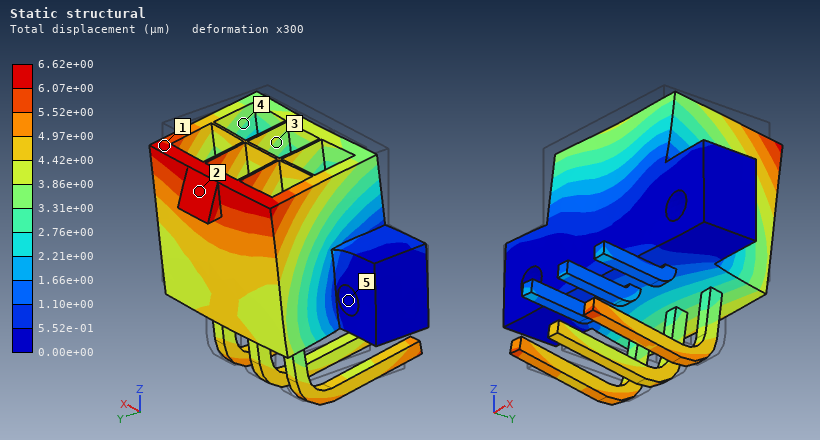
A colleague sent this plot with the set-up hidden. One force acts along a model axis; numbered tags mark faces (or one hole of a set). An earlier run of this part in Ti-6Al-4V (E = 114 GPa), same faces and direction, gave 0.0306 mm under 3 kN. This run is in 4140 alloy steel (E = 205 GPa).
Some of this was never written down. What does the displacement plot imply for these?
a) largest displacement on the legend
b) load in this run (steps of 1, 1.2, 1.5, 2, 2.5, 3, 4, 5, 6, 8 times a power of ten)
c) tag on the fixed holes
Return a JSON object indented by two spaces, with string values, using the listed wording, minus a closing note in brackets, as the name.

{
  "largest displacement on the legend": "6.62e+00 µm",
  "load in this run": "1.2 kN",
  "tag on the fixed holes": "5"
}
